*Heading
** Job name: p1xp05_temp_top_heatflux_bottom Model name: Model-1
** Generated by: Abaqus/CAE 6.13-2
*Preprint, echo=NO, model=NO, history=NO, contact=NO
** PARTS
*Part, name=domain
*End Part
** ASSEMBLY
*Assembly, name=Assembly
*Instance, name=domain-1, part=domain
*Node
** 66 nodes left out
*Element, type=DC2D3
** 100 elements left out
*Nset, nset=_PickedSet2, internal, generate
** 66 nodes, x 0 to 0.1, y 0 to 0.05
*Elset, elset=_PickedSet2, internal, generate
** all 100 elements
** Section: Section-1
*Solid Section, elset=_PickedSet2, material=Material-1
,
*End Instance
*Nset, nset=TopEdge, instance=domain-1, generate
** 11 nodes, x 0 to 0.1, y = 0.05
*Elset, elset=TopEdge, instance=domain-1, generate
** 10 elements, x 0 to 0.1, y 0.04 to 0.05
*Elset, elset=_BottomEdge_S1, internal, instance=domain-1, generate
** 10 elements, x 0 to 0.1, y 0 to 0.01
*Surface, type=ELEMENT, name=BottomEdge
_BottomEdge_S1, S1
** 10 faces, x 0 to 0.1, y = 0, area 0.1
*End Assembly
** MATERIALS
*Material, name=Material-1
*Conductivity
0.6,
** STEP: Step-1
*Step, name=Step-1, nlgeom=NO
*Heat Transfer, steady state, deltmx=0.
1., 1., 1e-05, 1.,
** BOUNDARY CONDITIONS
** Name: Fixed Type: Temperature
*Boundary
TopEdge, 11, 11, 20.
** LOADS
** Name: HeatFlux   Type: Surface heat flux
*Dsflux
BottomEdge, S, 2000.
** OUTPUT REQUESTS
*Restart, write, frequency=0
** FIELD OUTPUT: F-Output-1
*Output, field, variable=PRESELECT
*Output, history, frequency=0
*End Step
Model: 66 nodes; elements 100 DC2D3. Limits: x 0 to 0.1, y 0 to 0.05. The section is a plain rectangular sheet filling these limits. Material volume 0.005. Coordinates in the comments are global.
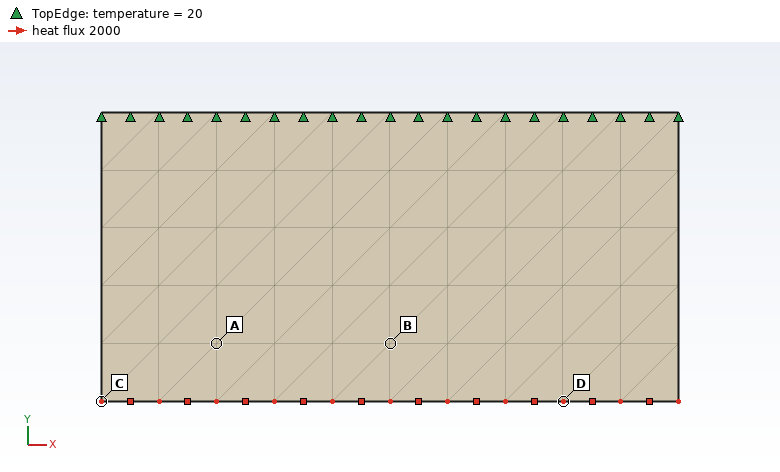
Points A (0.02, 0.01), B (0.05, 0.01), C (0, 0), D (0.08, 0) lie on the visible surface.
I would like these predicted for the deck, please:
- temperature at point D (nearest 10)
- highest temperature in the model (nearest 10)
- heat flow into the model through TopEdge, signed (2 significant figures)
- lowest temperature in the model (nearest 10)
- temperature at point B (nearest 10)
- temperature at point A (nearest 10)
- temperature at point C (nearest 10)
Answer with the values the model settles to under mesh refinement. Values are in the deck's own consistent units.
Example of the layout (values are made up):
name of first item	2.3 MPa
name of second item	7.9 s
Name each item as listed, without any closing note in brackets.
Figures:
temperature at point D	190
highest temperature in the model	190
heat flow into the model through TopEdge, signed	-200
lowest temperature in the model	20
temperature at point B	150
temperature at point A	150
temperature at point C	190
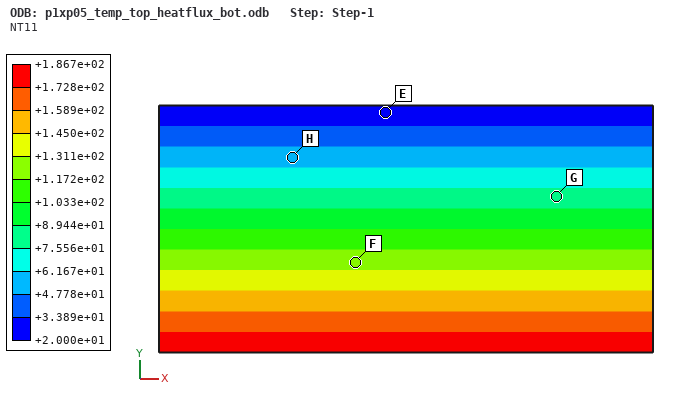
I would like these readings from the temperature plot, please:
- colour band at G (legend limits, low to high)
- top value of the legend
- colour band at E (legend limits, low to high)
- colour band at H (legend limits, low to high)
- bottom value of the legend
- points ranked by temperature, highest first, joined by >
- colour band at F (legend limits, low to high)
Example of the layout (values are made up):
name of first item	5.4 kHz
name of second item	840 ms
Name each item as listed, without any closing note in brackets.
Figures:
colour band at G	+7.556e+01 to +8.944e+01
top value of the legend	+1.867e+02
colour band at E	+2.000e+01 to +3.389e+01
colour band at H	+4.778e+01 to +6.167e+01
bottom value of the legend	+2.000e+01
points ranked by temperature, highest first, joined by >	F > G > H > E
colour band at F	+1.172e+02 to +1.311e+02
